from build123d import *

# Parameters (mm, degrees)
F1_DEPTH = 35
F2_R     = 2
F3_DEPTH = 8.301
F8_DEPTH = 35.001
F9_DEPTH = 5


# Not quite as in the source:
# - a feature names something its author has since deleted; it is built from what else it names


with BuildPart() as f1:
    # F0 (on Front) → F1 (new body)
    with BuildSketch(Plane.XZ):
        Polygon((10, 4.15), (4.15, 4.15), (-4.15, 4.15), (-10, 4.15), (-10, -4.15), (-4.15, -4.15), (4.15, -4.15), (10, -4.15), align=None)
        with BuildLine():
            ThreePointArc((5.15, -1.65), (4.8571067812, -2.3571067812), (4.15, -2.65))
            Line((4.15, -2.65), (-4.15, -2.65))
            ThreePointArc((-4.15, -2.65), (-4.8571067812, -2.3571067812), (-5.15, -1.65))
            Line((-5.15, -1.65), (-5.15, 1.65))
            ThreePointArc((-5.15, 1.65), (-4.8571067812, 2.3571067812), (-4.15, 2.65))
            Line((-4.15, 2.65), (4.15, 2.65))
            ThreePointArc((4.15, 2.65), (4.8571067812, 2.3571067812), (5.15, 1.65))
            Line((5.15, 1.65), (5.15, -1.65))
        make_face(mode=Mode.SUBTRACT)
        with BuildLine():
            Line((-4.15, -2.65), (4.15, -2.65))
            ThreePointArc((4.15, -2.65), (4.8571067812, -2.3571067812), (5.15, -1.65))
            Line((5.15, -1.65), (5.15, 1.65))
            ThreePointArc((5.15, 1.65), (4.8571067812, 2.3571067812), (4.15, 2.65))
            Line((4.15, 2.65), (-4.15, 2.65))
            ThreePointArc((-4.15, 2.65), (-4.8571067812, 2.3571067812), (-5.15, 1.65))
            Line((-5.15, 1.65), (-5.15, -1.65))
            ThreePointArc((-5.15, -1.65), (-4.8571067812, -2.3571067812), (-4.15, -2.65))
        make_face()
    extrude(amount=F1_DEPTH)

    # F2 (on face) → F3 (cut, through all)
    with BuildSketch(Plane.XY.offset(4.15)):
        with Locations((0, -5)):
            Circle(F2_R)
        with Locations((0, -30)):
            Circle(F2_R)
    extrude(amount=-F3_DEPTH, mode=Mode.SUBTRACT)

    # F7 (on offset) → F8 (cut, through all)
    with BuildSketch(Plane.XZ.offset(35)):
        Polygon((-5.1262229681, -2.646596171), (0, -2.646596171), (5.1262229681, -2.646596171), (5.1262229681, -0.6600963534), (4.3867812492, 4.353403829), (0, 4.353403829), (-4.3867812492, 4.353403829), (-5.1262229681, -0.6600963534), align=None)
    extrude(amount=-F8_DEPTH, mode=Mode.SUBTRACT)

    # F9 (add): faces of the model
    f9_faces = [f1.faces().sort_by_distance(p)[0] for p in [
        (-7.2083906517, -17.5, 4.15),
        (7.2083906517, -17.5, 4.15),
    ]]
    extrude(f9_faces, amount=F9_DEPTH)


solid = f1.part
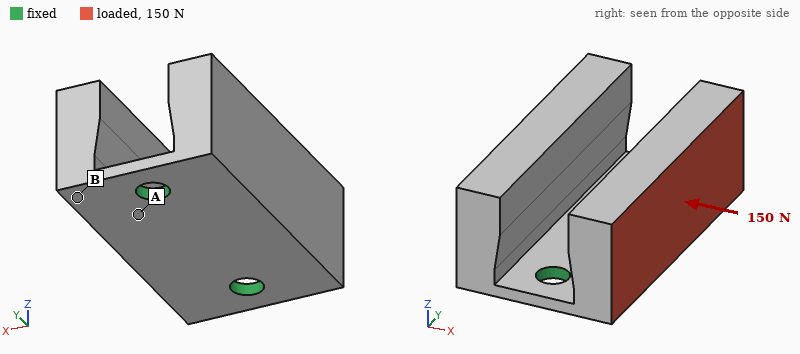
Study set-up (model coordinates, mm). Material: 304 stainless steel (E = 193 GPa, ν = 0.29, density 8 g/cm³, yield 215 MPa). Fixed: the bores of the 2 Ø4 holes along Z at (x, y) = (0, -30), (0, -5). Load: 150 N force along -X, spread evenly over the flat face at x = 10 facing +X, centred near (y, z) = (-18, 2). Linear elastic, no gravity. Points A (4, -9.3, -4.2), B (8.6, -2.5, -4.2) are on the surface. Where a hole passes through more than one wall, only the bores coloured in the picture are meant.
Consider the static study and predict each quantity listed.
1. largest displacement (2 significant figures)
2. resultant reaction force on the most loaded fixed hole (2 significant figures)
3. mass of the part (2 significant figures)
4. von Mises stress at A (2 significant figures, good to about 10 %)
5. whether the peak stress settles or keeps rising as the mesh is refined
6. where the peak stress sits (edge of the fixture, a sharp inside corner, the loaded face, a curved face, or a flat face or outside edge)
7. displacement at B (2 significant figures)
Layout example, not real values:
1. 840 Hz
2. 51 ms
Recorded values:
1. 32 µm
2. 75 N
3. 43 g
4. 55 MPa
5. keeps rising
6. edge of the fixture
7. 12 µm
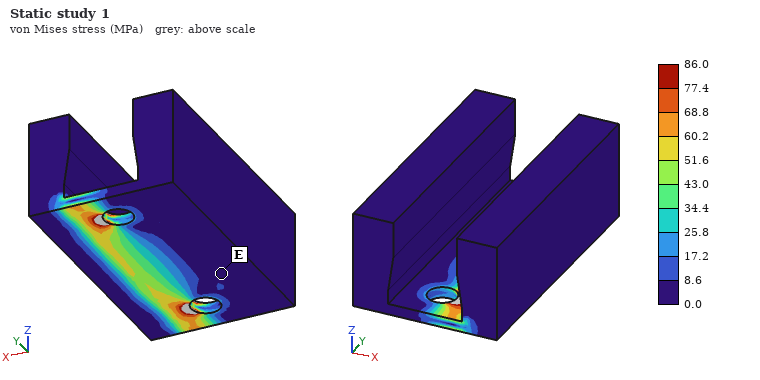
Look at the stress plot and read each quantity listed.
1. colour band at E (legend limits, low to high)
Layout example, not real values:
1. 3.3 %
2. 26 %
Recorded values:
1. 0.0 to 8.6 MPa
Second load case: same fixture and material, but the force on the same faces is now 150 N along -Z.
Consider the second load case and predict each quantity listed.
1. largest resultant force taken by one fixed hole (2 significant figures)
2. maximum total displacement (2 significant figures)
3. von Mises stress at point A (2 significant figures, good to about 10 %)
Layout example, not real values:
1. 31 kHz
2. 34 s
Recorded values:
1. 75 N
2. 37 µm
3. 58 MPa
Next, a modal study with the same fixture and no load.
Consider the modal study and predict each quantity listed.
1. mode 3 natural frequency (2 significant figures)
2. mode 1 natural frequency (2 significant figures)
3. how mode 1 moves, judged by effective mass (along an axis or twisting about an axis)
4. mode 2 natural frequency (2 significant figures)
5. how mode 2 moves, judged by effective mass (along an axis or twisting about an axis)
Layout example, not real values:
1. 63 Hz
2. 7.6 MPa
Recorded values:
1. 9600 Hz
2. 2600 Hz
3. along X
4. 2700 Hz
5. along Z
